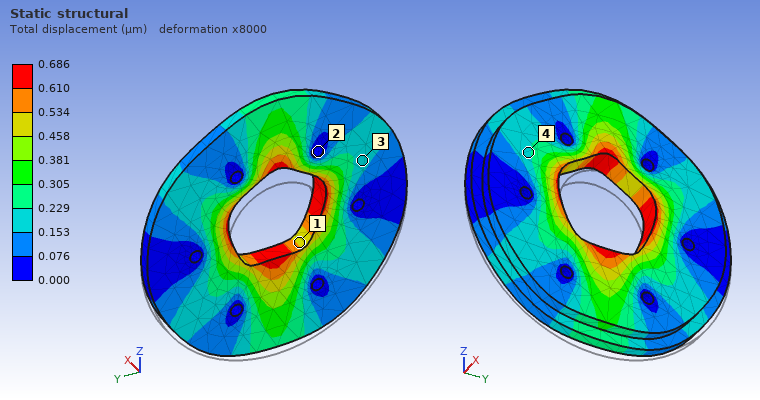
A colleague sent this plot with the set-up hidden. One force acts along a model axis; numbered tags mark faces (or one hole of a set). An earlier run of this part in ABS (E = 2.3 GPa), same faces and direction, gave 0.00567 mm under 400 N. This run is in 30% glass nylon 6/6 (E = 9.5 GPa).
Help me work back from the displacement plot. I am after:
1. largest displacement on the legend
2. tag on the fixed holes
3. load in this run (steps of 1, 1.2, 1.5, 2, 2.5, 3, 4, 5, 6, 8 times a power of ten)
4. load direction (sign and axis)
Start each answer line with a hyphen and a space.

- 0.686 µm
- 2
- 200 N
- +Z
